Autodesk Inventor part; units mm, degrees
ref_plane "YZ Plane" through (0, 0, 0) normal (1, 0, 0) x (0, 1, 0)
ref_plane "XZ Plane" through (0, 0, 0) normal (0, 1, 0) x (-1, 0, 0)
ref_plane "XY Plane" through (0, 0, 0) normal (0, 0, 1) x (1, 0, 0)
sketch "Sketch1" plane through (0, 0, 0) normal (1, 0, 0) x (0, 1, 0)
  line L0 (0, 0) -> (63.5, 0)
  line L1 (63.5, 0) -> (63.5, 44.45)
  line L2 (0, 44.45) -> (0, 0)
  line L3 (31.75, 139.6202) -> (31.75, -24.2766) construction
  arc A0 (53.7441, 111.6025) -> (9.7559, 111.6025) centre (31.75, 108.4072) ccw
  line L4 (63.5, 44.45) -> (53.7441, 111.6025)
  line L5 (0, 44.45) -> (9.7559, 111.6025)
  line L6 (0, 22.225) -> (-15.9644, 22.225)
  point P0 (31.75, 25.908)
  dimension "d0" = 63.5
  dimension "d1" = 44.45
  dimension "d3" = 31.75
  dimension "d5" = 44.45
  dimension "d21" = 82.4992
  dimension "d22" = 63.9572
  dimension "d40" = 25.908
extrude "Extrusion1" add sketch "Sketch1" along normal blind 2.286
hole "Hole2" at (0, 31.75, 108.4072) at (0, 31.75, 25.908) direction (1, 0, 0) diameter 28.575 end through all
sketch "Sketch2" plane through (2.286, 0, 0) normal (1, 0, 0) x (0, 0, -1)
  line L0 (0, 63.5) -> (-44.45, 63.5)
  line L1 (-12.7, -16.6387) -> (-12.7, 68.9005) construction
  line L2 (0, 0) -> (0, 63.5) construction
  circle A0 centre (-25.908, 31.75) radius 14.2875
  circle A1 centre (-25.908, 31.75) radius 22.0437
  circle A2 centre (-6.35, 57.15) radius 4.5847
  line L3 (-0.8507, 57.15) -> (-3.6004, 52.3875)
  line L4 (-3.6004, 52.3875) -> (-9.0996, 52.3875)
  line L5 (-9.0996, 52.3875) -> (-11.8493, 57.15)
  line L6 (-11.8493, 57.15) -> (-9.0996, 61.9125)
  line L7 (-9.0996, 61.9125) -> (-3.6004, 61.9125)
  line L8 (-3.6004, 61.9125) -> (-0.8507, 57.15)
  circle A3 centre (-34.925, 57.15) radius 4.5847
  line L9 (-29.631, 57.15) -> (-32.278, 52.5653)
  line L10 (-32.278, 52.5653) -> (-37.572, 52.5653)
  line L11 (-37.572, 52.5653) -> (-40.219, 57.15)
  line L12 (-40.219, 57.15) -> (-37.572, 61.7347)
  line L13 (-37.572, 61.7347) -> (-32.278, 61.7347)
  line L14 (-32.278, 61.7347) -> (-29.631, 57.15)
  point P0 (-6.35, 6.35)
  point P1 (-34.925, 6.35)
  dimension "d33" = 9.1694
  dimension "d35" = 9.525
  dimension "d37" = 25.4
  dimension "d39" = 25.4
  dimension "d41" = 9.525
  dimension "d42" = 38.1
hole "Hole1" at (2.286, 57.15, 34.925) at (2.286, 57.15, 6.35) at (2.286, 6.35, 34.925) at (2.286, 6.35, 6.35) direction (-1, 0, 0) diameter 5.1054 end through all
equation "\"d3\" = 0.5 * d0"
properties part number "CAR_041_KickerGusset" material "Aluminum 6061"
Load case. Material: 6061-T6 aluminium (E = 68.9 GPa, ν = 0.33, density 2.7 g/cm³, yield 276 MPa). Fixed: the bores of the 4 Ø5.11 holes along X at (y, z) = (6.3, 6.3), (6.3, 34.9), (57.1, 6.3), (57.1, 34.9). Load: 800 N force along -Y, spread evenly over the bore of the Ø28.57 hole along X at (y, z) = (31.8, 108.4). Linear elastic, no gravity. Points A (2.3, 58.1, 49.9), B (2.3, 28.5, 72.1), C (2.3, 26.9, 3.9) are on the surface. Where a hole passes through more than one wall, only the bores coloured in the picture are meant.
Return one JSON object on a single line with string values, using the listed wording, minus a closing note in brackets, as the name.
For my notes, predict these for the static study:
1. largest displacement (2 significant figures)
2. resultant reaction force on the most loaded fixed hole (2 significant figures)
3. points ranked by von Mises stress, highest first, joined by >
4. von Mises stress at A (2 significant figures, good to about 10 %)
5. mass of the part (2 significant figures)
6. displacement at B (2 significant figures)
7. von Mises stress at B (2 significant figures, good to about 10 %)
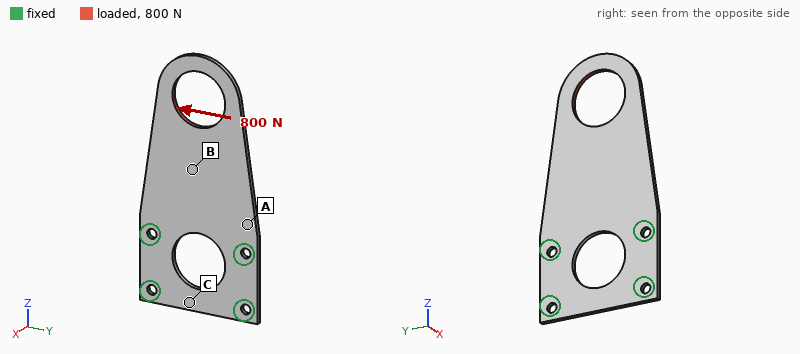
{"largest displacement": "0.12 mm", "resultant reaction force on the most loaded fixed hole": "1.1 kN", "points ranked by von Mises stress, highest first, joined by >": "A > B > C", "von Mises stress at A": "30 MPa", "mass of the part": "35 g", "displacement at B": "0.020 mm", "von Mises stress at B": "16 MPa"}
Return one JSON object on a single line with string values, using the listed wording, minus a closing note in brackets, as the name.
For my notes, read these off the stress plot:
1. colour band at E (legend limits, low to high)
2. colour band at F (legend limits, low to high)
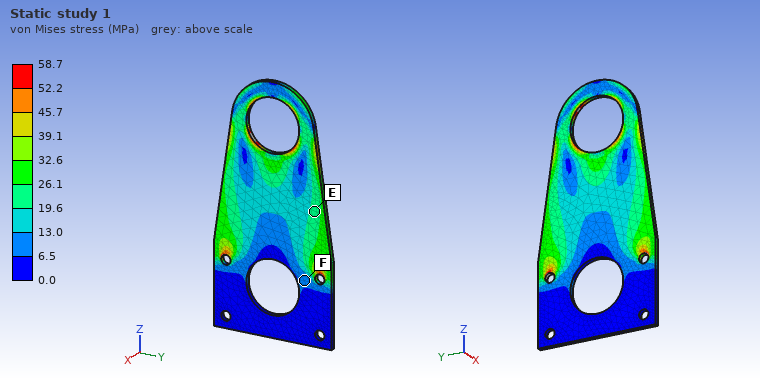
{"colour band at E": "19.6 to 26.1 MPa", "colour band at F": "6.5 to 13.0 MPa"}
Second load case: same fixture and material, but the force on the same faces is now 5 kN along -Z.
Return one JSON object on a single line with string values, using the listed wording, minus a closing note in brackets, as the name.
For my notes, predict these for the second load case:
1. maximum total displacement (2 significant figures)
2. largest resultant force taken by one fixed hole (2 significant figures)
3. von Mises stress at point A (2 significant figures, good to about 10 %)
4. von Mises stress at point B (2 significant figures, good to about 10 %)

{"maximum total displacement": "0.12 mm", "largest resultant force taken by one fixed hole": "2.3 kN", "von Mises stress at point A": "52 MPa", "von Mises stress at point B": "25 MPa"}
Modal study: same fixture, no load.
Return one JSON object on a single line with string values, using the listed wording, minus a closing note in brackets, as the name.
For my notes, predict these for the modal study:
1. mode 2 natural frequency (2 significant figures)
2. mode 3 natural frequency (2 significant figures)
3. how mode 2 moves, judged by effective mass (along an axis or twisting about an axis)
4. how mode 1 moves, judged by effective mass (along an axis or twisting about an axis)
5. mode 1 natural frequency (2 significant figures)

{"mode 2 natural frequency": "1100 Hz", "mode 3 natural frequency": "1300 Hz", "how mode 2 moves, judged by effective mass": "twisting about Z", "how mode 1 moves, judged by effective mass": "along X", "mode 1 natural frequency": "290 Hz"}
